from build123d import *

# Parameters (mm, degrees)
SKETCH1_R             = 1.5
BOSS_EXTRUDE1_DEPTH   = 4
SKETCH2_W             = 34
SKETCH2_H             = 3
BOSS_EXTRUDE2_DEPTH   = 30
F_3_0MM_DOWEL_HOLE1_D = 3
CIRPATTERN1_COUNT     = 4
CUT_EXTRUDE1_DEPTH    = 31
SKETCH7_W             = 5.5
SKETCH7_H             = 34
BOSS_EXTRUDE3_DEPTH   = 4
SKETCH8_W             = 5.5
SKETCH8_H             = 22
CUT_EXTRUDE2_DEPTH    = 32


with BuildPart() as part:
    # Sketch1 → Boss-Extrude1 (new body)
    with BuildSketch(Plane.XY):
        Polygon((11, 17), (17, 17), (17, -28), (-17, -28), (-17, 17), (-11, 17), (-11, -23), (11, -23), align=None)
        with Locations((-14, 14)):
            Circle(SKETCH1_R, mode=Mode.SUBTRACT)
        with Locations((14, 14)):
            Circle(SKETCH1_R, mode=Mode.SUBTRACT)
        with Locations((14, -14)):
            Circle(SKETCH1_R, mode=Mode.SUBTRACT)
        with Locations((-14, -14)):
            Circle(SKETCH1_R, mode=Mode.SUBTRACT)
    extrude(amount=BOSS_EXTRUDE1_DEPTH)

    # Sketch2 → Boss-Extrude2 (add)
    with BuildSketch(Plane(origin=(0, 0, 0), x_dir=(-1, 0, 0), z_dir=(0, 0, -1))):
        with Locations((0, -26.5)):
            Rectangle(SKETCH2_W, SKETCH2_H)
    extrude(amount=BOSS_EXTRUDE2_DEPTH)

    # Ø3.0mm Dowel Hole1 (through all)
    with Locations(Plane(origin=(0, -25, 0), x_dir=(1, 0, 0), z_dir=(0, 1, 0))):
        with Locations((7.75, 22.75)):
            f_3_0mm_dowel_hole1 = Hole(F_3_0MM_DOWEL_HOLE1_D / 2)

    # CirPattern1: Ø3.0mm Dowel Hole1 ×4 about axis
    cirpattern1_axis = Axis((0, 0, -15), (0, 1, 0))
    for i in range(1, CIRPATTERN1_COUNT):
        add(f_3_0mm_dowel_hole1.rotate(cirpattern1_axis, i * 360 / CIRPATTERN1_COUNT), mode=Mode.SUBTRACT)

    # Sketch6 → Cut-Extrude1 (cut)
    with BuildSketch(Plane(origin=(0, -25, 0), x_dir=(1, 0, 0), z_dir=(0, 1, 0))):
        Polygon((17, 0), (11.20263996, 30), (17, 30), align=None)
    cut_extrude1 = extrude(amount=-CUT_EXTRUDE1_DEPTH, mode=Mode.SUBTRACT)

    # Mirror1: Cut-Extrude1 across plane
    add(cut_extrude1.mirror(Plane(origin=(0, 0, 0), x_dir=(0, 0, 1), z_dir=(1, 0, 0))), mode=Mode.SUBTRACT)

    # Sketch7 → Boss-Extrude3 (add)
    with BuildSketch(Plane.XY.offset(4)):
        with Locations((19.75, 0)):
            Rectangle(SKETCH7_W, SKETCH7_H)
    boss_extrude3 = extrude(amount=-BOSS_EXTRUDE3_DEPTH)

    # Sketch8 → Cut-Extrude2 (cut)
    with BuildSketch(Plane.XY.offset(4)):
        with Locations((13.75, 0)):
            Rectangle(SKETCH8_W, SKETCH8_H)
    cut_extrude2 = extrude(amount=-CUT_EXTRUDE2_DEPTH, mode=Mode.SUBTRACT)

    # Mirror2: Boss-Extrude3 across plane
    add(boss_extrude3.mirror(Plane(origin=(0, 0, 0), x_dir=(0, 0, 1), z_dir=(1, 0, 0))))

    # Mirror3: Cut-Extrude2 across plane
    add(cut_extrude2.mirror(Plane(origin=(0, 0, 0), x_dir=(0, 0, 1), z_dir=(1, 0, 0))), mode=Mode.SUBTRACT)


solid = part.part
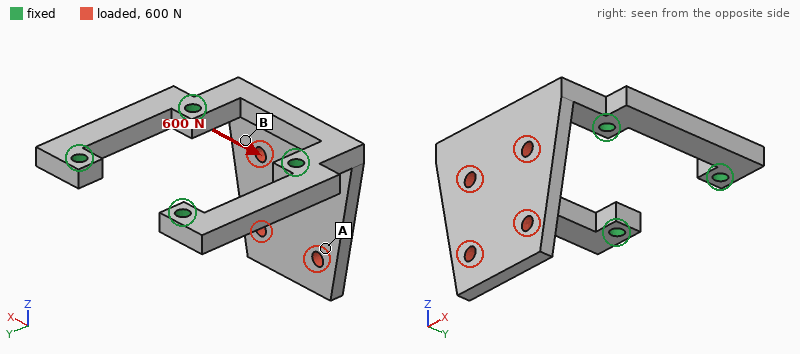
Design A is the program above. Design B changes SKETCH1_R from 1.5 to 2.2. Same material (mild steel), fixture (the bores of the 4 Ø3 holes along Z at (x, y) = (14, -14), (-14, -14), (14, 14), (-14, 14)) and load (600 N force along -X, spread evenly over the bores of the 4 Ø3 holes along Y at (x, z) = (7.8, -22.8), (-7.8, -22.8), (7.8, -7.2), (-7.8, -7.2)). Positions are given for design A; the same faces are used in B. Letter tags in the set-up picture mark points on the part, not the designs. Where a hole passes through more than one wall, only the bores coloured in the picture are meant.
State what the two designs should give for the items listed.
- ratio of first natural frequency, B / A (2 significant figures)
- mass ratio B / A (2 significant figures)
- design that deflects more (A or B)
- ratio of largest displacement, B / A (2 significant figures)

1.0
0.98
A
0.86
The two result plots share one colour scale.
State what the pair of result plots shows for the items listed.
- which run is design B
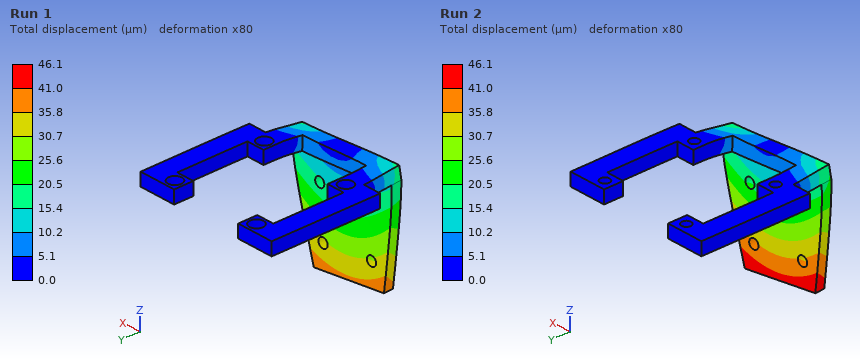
Run 1
